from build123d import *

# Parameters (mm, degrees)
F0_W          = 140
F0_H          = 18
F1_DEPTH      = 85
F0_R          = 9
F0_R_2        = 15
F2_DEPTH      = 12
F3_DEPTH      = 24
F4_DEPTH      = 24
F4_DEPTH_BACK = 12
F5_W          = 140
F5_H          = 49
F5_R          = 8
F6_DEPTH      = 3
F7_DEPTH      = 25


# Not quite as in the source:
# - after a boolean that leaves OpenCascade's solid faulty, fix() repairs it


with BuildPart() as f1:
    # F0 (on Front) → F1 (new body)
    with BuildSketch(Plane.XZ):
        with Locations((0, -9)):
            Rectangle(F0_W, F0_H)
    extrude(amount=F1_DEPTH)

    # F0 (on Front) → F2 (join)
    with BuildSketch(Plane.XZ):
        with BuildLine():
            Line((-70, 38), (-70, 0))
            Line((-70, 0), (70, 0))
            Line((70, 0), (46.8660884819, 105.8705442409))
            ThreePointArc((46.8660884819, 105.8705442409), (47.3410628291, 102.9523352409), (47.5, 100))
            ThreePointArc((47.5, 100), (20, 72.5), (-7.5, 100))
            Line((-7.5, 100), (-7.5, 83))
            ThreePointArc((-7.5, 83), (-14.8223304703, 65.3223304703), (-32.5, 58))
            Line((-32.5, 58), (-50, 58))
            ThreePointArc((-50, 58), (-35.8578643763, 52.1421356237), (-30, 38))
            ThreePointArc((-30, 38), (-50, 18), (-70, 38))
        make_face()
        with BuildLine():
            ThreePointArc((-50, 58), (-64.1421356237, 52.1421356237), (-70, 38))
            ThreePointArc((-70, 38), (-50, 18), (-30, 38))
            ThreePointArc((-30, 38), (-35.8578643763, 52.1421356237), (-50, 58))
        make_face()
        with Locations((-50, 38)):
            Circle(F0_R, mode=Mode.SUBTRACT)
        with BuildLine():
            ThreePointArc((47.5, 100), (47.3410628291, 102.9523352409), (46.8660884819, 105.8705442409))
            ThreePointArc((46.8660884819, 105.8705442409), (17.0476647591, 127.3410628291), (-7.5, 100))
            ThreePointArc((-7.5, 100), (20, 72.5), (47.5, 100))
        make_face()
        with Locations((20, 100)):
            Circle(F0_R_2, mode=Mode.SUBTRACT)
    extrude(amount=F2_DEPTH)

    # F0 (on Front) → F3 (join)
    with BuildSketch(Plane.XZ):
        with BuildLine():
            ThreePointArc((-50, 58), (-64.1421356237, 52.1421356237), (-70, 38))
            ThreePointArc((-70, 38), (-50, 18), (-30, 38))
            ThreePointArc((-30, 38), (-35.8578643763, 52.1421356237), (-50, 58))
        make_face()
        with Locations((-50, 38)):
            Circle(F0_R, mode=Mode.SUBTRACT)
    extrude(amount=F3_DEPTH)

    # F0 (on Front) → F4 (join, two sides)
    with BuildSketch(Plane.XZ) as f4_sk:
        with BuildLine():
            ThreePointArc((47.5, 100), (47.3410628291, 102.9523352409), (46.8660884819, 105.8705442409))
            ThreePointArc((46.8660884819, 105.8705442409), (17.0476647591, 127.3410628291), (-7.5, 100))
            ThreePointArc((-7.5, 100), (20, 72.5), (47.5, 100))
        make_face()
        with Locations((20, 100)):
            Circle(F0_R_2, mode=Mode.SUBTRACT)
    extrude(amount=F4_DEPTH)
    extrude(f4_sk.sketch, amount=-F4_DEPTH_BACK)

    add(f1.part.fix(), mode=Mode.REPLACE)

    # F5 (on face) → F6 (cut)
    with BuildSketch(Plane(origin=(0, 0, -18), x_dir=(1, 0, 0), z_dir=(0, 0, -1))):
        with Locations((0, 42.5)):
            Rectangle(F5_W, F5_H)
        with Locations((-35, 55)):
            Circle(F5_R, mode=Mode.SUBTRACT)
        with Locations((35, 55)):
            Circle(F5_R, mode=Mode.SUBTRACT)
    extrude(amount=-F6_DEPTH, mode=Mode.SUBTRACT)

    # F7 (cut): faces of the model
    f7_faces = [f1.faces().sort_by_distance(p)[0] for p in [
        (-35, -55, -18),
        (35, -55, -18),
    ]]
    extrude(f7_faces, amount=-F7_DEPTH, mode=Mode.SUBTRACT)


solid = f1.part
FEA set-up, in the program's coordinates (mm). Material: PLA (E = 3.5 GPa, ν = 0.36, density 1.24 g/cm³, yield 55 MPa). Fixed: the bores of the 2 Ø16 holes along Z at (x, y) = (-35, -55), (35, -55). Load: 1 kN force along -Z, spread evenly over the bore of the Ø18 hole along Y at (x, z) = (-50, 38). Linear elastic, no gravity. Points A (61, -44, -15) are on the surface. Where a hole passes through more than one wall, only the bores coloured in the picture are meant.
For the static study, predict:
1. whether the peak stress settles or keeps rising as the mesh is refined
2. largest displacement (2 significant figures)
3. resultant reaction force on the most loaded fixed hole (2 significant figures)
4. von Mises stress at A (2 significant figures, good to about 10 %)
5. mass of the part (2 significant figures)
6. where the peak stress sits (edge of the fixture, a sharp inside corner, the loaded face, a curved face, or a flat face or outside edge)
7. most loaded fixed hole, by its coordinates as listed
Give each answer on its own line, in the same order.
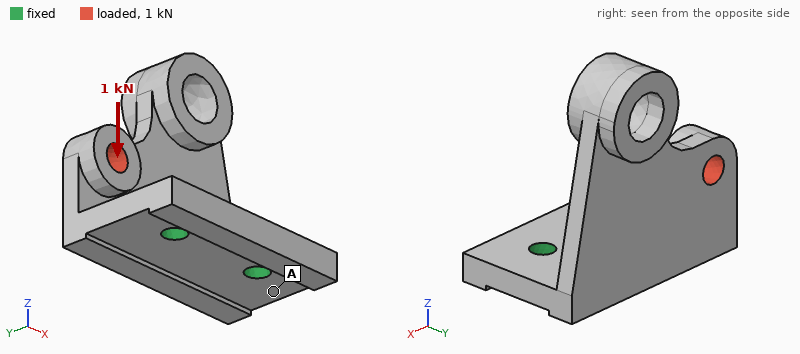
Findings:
keeps rising
0.77 mm
1.1 kN
1.6 MPa
450 g
edge of the fixture
(-35, -55)
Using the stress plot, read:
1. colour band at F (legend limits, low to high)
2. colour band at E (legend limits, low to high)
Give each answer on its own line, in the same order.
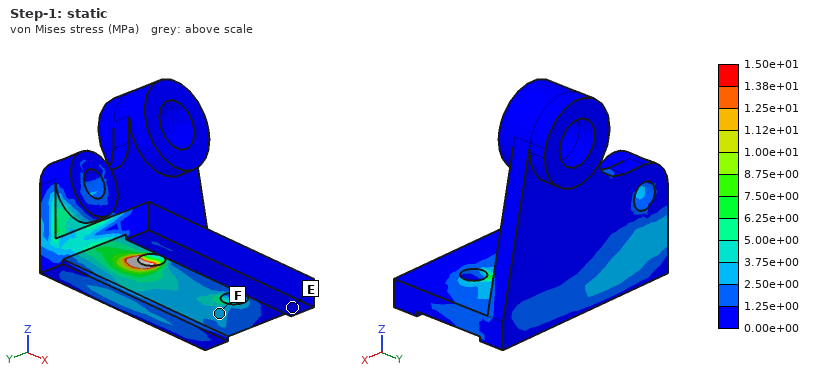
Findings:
2.50e+00 to 3.75e+00 MPa
0.00e+00 to 1.25e+00 MPa
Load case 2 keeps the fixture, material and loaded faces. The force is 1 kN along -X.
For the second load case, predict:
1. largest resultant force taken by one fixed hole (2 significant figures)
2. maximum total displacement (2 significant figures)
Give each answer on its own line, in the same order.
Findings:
890 N
0.65 mm
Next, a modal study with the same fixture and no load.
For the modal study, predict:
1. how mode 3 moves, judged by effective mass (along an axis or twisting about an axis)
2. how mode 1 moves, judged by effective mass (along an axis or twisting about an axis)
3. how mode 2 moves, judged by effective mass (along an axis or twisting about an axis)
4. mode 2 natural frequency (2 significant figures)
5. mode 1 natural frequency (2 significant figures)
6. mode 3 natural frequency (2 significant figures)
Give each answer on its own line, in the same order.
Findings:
along Z
along Y
along X
410 Hz
160 Hz
590 Hz
